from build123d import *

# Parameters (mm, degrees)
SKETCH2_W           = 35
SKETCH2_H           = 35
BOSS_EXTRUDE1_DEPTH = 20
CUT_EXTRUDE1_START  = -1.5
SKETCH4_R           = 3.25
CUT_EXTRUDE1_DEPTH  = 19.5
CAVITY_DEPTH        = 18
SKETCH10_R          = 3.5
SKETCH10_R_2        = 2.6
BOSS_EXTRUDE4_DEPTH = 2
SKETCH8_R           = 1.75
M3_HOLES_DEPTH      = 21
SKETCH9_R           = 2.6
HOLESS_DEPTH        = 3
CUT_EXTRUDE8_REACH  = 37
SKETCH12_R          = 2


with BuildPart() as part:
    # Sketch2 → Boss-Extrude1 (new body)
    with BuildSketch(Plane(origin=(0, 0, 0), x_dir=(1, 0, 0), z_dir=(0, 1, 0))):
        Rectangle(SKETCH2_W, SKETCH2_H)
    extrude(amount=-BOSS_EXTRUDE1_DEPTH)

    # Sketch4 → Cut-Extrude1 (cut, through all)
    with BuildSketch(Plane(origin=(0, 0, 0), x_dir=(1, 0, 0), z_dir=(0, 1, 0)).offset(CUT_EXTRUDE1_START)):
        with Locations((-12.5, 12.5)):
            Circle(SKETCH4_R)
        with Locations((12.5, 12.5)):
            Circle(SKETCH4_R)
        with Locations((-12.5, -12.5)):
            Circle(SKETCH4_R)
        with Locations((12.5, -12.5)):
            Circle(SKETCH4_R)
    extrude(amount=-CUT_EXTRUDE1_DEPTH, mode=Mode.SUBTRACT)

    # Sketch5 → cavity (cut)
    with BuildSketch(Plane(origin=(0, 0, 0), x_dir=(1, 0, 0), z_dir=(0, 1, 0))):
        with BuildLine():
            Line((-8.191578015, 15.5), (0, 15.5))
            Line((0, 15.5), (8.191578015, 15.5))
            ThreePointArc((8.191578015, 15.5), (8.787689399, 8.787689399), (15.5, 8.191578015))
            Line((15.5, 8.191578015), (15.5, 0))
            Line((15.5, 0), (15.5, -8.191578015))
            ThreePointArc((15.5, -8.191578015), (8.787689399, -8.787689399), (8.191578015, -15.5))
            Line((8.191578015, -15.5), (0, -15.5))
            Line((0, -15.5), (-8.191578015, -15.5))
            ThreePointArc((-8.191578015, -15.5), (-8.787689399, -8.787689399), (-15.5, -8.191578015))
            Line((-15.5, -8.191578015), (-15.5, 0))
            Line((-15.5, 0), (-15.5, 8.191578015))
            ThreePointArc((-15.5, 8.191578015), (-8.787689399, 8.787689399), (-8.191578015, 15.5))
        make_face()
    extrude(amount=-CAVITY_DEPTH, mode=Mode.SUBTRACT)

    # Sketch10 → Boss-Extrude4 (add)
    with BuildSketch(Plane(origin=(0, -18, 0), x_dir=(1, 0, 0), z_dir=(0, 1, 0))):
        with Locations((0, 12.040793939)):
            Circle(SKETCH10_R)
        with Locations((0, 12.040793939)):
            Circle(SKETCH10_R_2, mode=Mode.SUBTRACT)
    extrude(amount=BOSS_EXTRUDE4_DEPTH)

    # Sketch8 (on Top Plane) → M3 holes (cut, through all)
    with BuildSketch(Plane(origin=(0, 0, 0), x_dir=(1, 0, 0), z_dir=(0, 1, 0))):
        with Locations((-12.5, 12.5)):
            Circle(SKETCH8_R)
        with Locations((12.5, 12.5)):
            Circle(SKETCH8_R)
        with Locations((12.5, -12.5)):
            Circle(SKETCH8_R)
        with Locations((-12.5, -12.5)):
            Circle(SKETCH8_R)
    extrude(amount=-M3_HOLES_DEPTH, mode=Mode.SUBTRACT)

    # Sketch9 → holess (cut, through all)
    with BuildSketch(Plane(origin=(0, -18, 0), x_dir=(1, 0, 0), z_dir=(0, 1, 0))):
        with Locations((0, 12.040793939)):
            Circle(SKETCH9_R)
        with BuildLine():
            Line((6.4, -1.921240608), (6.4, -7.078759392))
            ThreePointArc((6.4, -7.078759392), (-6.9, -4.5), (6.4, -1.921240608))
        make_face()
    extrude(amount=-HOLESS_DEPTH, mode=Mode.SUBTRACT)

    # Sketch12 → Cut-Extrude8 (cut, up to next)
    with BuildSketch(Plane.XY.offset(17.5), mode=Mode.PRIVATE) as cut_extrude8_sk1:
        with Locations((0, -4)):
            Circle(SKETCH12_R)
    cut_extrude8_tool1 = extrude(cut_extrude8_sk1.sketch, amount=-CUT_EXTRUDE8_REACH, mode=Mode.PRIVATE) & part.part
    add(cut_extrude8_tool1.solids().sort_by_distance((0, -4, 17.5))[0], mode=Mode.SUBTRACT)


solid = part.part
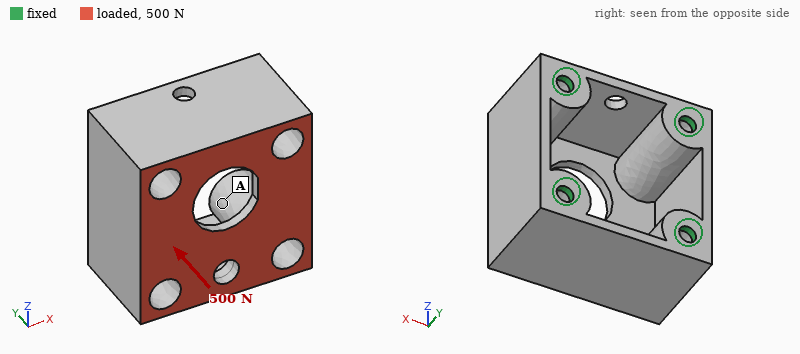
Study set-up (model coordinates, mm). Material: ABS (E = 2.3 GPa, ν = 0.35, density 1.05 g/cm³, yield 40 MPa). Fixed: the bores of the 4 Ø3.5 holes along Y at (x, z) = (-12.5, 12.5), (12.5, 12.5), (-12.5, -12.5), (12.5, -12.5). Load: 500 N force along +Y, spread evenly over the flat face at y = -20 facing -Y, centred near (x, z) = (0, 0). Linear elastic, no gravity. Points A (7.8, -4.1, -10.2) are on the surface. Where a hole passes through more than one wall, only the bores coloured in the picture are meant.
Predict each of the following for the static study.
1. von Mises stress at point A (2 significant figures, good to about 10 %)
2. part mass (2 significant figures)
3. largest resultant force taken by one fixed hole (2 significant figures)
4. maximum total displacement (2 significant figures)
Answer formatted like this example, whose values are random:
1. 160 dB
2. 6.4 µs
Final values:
1. 2.8 MPa
2. 9.1 g
3. 130 N
4. 0.35 mm
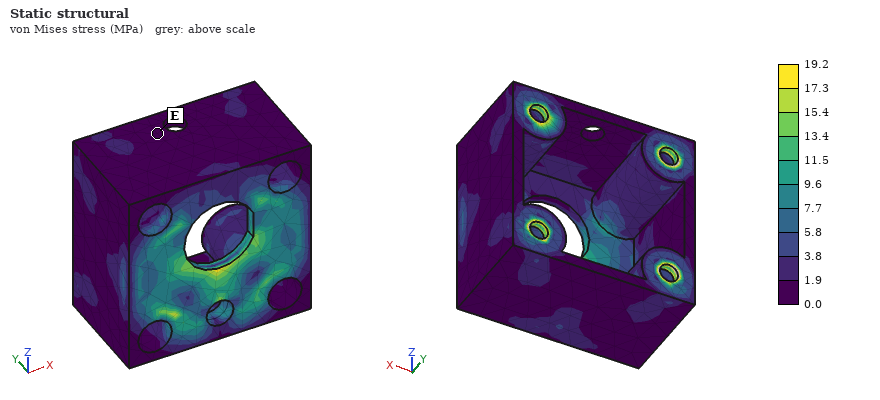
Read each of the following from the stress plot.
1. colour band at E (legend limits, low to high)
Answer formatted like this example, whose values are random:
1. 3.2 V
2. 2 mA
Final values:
1. 0.0 to 1.9 MPa
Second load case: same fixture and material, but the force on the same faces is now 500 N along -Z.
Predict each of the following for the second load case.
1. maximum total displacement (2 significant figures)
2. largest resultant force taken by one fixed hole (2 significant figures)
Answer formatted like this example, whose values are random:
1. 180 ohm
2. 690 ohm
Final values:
1. 0.26 mm
2. 220 N
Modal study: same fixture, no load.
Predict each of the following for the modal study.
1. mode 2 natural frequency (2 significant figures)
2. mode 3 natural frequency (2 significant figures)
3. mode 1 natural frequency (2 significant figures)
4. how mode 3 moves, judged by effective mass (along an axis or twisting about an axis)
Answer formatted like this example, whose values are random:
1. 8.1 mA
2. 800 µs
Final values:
1. 3600 Hz
2. 5700 Hz
3. 3500 Hz
4. along Y
